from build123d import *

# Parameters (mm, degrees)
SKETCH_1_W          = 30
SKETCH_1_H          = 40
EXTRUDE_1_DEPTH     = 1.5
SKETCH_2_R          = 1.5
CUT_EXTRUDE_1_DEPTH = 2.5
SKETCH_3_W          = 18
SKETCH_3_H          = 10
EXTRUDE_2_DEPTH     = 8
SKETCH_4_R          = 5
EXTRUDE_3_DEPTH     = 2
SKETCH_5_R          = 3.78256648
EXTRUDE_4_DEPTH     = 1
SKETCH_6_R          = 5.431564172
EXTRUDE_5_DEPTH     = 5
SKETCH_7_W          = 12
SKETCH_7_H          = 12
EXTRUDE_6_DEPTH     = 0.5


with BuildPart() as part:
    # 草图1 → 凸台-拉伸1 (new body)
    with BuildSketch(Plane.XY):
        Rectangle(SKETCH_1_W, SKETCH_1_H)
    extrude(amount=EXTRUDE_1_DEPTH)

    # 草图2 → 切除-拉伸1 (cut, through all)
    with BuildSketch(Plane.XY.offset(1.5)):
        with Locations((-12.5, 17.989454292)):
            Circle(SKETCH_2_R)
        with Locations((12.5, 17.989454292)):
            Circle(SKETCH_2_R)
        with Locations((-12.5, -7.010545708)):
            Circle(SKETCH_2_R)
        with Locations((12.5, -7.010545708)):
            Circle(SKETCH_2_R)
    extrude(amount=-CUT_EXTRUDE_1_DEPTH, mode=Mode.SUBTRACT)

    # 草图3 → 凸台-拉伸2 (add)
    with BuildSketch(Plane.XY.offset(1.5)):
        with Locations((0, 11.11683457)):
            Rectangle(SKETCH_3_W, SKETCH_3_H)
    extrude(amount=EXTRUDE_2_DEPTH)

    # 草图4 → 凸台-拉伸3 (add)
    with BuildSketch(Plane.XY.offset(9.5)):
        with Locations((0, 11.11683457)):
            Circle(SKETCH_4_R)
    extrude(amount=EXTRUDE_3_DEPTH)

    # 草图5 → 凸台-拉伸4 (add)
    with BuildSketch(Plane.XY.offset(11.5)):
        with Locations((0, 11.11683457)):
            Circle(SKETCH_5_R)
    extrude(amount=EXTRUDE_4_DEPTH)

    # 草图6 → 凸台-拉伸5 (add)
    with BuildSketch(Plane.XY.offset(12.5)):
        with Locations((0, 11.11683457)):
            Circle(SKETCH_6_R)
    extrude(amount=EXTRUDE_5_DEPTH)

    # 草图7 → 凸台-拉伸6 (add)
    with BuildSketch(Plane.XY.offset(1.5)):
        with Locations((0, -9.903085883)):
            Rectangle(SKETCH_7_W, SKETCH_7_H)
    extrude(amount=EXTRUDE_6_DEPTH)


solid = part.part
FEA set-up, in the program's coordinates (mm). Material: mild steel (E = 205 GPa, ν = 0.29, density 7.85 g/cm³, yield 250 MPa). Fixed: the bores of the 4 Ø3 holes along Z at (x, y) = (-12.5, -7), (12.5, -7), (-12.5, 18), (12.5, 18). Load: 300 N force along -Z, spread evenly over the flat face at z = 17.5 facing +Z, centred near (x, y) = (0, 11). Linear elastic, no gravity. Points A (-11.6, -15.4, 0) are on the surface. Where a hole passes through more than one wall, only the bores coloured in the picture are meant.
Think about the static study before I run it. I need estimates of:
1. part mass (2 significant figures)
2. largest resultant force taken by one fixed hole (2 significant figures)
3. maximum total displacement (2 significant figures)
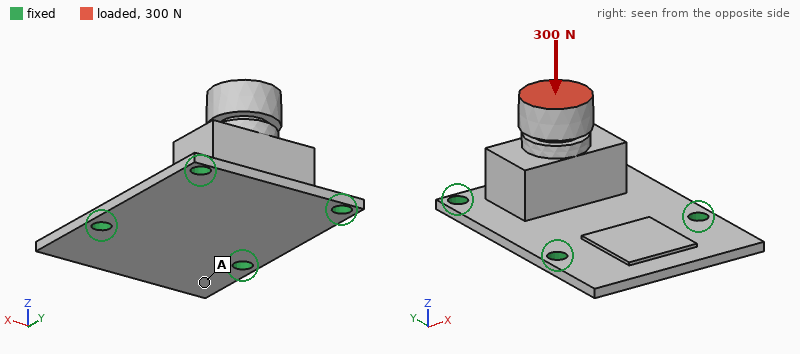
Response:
31 g
120 N
13 µm
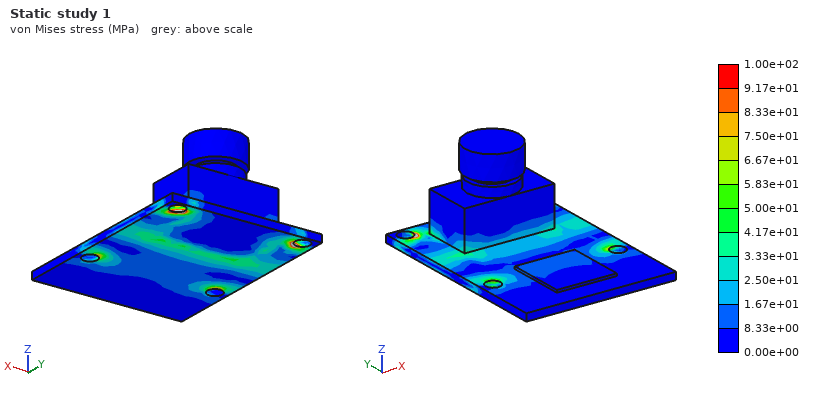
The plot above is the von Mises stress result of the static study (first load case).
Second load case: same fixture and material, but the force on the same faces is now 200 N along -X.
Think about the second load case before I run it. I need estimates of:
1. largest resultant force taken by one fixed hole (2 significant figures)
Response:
180 N
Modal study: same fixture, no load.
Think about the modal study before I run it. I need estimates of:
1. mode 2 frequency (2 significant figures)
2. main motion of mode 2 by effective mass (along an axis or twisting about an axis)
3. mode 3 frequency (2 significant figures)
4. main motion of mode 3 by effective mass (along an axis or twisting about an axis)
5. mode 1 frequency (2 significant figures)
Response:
6900 Hz
along Z
11 kHz
along X
4900 Hz
